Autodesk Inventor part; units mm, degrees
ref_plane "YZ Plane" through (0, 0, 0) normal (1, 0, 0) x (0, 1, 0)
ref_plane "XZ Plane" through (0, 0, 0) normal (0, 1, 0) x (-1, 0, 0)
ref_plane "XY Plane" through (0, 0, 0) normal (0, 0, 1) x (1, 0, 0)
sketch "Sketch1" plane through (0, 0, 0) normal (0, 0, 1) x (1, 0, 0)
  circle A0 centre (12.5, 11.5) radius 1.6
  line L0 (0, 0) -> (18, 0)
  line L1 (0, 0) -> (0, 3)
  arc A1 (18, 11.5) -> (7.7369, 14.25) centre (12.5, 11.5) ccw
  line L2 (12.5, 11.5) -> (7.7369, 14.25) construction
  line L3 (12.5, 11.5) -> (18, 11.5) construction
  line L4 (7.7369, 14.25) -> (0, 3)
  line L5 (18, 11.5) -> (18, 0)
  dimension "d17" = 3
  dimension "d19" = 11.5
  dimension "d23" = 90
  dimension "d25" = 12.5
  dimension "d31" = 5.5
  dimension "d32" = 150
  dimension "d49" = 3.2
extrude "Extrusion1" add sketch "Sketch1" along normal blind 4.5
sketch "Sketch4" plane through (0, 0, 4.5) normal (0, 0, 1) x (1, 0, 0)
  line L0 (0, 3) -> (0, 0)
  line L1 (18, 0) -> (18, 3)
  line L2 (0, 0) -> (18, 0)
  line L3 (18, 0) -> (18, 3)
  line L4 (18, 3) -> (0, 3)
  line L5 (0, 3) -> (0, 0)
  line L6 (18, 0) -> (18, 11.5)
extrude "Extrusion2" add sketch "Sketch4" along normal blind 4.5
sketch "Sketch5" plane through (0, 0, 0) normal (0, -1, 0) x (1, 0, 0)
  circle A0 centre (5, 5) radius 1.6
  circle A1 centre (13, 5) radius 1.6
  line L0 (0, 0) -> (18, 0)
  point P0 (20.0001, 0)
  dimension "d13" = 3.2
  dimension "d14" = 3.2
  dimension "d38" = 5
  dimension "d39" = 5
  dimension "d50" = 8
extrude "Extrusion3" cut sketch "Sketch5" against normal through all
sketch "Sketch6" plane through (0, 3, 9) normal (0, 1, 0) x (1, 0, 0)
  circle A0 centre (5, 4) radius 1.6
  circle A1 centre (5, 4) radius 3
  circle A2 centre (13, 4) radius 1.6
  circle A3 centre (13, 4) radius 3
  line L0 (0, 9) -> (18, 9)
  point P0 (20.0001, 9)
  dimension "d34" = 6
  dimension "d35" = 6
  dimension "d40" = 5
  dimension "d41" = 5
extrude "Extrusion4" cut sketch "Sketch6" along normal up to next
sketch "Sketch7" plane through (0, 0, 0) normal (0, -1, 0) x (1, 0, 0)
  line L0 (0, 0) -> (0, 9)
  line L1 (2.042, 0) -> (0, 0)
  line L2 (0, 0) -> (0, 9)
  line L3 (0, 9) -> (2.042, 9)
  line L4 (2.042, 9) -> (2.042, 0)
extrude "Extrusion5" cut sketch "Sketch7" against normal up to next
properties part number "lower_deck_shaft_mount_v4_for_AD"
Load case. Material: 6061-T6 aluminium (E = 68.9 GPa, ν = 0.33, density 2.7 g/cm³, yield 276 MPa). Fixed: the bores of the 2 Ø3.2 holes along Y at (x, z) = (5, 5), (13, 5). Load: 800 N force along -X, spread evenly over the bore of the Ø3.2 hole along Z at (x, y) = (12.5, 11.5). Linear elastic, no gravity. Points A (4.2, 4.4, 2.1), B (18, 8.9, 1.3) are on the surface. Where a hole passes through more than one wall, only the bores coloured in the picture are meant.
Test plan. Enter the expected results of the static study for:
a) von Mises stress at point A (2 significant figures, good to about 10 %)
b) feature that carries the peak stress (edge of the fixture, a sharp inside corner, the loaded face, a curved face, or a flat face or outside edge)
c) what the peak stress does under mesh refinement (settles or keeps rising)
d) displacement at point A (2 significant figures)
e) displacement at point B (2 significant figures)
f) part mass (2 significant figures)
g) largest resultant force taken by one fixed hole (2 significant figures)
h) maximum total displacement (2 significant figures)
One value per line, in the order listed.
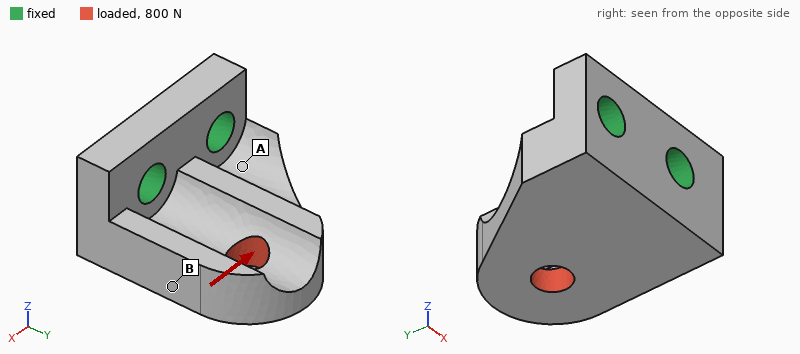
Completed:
100 MPa
edge of the fixture
keeps rising
10 µm
28 µm
2.5 g
880 N
46 µm
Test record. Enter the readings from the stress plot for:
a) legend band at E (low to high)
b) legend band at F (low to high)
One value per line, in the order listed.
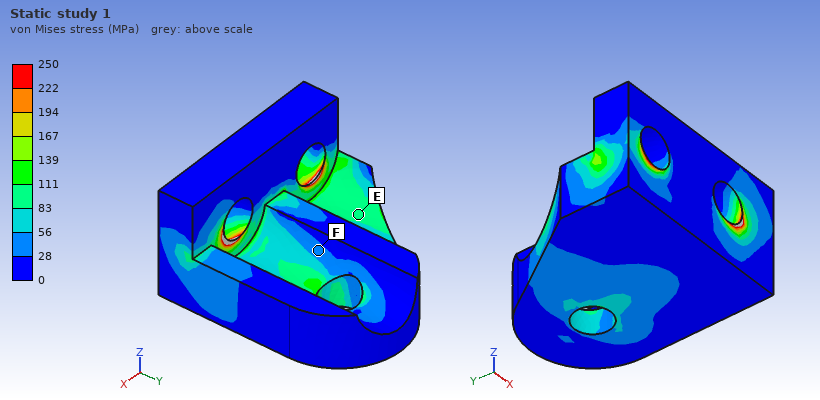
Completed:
83 to 111 MPa
28 to 56 MPa
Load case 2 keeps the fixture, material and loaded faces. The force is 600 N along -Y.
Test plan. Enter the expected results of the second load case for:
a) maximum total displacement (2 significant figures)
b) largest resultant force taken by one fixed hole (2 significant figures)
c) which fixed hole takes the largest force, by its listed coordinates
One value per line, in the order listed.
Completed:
33 µm
490 N
(13, 5)
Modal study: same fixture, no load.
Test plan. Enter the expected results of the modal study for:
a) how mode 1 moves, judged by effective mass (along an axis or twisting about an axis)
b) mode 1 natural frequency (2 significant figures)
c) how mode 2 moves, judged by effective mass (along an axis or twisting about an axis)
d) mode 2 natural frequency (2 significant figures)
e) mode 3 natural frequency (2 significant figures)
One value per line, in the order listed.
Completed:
along Z
13 kHz
along X
24 kHz
34 kHz
